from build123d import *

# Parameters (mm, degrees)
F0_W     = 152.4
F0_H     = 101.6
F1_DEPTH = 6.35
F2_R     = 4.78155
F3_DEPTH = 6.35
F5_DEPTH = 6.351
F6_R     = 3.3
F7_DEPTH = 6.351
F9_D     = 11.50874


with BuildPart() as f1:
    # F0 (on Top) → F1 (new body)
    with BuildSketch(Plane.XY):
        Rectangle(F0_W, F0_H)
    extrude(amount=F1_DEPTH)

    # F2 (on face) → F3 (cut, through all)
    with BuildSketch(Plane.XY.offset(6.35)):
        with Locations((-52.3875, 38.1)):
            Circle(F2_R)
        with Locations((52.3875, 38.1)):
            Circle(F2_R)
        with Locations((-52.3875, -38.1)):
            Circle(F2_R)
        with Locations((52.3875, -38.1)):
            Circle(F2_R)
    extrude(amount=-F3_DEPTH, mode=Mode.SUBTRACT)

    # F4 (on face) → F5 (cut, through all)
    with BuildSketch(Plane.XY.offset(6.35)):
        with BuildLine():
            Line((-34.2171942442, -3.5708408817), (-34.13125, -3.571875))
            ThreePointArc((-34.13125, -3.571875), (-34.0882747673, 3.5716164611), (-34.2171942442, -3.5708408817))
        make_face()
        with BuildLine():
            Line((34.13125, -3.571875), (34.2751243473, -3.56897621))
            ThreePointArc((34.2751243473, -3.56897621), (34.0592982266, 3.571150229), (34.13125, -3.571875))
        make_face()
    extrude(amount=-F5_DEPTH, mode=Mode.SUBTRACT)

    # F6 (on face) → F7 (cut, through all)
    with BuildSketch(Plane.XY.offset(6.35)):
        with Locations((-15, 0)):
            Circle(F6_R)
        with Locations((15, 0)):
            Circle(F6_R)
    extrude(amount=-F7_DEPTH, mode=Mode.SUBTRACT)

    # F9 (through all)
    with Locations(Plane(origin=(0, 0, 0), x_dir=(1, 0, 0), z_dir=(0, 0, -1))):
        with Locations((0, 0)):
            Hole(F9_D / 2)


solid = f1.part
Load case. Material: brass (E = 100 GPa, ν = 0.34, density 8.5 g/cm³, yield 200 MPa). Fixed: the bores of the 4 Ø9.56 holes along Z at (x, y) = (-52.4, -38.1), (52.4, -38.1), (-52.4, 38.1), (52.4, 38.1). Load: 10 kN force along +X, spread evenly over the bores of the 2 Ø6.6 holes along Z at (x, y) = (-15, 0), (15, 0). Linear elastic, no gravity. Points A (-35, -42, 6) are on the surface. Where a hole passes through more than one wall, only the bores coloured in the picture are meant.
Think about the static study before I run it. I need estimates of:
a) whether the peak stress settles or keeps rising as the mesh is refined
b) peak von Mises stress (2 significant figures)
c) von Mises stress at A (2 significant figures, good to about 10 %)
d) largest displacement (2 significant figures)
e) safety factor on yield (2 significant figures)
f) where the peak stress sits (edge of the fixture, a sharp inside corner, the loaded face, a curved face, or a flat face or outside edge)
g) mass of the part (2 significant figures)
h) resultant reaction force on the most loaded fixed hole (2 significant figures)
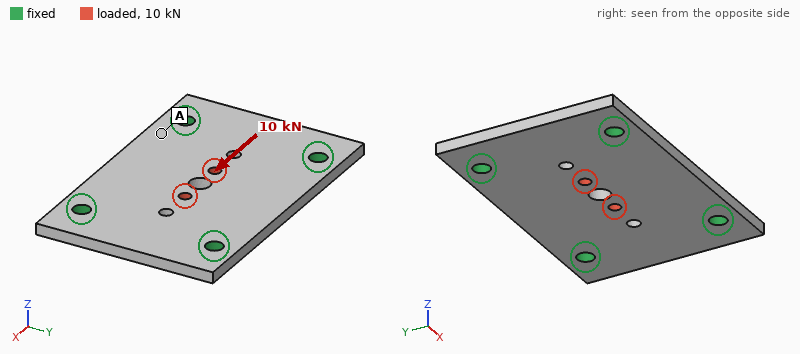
settles
70 MPa
7.9 MPa
12 µm
2.9
the loaded face
810 g
2.6 kN
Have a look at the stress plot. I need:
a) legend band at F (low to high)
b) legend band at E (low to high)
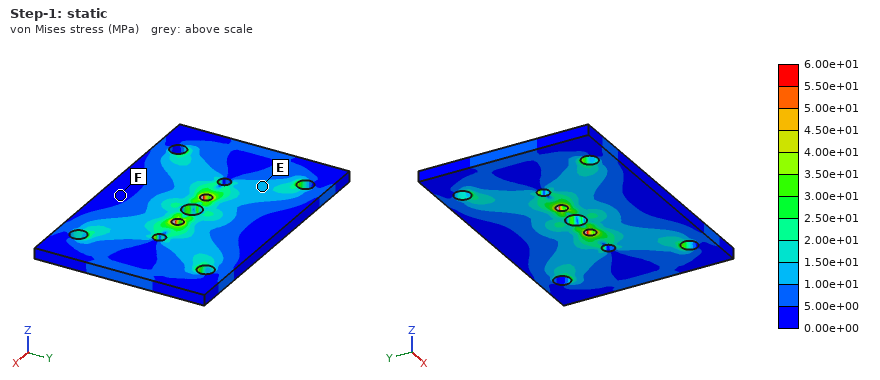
0.00e+00 to 5.00e+00 MPa
1.00e+01 to 1.50e+01 MPa
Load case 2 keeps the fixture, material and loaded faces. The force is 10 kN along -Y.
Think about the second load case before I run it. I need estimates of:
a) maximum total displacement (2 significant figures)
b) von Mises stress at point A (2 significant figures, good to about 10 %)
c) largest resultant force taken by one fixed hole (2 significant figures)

14 µm
9.7 MPa
2.9 kN
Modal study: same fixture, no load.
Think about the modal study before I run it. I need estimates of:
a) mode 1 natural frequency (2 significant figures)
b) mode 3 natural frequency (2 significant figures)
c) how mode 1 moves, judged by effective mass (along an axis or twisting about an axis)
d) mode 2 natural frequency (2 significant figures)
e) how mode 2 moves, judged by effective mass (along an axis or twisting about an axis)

1900 Hz
3400 Hz
along Z
2600 Hz
twisting about X
